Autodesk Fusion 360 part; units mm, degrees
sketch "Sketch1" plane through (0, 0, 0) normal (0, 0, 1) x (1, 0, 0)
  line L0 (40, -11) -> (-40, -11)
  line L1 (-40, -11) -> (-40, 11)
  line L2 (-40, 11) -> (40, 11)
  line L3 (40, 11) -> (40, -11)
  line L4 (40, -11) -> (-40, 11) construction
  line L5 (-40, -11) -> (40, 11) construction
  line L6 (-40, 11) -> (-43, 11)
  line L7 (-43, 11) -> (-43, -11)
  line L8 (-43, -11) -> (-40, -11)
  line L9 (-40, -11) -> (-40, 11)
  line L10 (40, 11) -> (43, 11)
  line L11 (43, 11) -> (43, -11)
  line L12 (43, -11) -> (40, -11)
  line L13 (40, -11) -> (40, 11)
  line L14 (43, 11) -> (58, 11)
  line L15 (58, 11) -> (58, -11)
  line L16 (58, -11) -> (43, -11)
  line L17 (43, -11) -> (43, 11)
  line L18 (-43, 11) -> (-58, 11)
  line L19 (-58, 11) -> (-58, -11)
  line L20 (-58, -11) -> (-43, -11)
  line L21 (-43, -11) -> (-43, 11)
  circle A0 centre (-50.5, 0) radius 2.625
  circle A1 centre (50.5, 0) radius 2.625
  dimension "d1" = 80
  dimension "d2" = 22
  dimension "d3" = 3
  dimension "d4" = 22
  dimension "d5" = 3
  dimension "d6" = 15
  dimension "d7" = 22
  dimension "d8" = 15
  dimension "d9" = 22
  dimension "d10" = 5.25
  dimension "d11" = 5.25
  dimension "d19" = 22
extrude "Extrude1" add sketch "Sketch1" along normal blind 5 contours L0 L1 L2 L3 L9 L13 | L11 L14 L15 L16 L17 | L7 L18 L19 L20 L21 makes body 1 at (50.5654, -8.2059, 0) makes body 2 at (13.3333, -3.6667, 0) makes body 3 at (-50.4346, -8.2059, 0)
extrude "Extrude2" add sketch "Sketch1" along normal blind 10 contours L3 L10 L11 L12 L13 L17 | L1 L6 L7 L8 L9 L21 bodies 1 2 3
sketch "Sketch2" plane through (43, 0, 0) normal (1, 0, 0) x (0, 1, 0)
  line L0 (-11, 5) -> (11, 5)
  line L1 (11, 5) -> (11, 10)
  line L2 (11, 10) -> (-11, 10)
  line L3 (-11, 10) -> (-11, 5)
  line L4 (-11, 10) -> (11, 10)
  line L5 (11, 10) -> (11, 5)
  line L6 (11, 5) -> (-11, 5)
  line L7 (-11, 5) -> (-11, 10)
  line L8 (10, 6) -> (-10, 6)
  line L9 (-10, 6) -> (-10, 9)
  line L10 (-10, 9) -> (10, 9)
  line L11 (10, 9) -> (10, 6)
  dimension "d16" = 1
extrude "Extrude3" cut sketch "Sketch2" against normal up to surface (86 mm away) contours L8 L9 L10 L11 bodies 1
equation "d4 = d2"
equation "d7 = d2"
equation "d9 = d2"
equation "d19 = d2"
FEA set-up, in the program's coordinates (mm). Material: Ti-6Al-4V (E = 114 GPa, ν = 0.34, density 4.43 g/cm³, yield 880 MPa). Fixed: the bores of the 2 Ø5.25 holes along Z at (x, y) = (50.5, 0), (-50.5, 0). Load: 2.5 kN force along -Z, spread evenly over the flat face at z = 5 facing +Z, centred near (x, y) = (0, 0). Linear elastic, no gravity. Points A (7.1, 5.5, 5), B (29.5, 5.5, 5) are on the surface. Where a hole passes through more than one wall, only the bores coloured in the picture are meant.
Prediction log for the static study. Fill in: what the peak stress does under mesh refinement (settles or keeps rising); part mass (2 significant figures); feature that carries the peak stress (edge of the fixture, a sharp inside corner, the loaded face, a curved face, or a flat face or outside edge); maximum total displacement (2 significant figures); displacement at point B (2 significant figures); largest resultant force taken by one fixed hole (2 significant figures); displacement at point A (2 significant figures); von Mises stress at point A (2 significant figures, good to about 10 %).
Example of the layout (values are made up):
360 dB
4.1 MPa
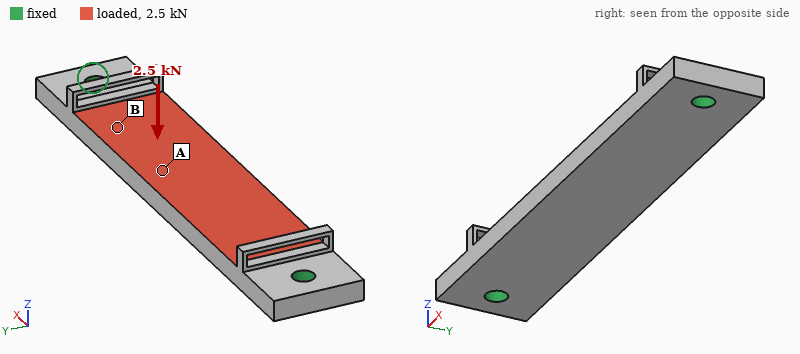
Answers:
keeps rising
57 g
edge of the fixture
0.31 mm
0.13 mm
1.3 kN
0.29 mm
130 MPa
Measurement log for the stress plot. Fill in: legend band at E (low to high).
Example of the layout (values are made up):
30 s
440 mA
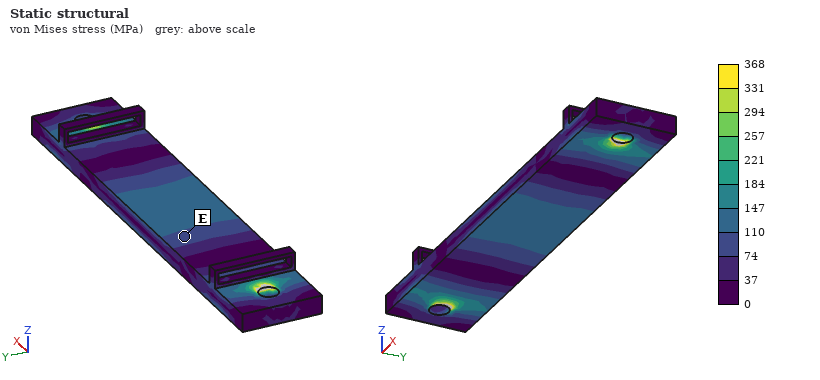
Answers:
74 to 110 MPa
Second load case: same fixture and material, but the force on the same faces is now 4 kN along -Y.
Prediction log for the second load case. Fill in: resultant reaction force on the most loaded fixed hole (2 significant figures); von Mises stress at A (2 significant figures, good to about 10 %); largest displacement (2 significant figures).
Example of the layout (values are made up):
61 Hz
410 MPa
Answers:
2.0 kN
37 MPa
93 µm
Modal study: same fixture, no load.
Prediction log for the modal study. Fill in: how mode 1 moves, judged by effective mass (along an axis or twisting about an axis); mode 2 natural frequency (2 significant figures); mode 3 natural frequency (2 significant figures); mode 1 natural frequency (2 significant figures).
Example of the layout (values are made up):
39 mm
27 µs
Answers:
along Z
6600 Hz
6600 Hz
2600 Hz
